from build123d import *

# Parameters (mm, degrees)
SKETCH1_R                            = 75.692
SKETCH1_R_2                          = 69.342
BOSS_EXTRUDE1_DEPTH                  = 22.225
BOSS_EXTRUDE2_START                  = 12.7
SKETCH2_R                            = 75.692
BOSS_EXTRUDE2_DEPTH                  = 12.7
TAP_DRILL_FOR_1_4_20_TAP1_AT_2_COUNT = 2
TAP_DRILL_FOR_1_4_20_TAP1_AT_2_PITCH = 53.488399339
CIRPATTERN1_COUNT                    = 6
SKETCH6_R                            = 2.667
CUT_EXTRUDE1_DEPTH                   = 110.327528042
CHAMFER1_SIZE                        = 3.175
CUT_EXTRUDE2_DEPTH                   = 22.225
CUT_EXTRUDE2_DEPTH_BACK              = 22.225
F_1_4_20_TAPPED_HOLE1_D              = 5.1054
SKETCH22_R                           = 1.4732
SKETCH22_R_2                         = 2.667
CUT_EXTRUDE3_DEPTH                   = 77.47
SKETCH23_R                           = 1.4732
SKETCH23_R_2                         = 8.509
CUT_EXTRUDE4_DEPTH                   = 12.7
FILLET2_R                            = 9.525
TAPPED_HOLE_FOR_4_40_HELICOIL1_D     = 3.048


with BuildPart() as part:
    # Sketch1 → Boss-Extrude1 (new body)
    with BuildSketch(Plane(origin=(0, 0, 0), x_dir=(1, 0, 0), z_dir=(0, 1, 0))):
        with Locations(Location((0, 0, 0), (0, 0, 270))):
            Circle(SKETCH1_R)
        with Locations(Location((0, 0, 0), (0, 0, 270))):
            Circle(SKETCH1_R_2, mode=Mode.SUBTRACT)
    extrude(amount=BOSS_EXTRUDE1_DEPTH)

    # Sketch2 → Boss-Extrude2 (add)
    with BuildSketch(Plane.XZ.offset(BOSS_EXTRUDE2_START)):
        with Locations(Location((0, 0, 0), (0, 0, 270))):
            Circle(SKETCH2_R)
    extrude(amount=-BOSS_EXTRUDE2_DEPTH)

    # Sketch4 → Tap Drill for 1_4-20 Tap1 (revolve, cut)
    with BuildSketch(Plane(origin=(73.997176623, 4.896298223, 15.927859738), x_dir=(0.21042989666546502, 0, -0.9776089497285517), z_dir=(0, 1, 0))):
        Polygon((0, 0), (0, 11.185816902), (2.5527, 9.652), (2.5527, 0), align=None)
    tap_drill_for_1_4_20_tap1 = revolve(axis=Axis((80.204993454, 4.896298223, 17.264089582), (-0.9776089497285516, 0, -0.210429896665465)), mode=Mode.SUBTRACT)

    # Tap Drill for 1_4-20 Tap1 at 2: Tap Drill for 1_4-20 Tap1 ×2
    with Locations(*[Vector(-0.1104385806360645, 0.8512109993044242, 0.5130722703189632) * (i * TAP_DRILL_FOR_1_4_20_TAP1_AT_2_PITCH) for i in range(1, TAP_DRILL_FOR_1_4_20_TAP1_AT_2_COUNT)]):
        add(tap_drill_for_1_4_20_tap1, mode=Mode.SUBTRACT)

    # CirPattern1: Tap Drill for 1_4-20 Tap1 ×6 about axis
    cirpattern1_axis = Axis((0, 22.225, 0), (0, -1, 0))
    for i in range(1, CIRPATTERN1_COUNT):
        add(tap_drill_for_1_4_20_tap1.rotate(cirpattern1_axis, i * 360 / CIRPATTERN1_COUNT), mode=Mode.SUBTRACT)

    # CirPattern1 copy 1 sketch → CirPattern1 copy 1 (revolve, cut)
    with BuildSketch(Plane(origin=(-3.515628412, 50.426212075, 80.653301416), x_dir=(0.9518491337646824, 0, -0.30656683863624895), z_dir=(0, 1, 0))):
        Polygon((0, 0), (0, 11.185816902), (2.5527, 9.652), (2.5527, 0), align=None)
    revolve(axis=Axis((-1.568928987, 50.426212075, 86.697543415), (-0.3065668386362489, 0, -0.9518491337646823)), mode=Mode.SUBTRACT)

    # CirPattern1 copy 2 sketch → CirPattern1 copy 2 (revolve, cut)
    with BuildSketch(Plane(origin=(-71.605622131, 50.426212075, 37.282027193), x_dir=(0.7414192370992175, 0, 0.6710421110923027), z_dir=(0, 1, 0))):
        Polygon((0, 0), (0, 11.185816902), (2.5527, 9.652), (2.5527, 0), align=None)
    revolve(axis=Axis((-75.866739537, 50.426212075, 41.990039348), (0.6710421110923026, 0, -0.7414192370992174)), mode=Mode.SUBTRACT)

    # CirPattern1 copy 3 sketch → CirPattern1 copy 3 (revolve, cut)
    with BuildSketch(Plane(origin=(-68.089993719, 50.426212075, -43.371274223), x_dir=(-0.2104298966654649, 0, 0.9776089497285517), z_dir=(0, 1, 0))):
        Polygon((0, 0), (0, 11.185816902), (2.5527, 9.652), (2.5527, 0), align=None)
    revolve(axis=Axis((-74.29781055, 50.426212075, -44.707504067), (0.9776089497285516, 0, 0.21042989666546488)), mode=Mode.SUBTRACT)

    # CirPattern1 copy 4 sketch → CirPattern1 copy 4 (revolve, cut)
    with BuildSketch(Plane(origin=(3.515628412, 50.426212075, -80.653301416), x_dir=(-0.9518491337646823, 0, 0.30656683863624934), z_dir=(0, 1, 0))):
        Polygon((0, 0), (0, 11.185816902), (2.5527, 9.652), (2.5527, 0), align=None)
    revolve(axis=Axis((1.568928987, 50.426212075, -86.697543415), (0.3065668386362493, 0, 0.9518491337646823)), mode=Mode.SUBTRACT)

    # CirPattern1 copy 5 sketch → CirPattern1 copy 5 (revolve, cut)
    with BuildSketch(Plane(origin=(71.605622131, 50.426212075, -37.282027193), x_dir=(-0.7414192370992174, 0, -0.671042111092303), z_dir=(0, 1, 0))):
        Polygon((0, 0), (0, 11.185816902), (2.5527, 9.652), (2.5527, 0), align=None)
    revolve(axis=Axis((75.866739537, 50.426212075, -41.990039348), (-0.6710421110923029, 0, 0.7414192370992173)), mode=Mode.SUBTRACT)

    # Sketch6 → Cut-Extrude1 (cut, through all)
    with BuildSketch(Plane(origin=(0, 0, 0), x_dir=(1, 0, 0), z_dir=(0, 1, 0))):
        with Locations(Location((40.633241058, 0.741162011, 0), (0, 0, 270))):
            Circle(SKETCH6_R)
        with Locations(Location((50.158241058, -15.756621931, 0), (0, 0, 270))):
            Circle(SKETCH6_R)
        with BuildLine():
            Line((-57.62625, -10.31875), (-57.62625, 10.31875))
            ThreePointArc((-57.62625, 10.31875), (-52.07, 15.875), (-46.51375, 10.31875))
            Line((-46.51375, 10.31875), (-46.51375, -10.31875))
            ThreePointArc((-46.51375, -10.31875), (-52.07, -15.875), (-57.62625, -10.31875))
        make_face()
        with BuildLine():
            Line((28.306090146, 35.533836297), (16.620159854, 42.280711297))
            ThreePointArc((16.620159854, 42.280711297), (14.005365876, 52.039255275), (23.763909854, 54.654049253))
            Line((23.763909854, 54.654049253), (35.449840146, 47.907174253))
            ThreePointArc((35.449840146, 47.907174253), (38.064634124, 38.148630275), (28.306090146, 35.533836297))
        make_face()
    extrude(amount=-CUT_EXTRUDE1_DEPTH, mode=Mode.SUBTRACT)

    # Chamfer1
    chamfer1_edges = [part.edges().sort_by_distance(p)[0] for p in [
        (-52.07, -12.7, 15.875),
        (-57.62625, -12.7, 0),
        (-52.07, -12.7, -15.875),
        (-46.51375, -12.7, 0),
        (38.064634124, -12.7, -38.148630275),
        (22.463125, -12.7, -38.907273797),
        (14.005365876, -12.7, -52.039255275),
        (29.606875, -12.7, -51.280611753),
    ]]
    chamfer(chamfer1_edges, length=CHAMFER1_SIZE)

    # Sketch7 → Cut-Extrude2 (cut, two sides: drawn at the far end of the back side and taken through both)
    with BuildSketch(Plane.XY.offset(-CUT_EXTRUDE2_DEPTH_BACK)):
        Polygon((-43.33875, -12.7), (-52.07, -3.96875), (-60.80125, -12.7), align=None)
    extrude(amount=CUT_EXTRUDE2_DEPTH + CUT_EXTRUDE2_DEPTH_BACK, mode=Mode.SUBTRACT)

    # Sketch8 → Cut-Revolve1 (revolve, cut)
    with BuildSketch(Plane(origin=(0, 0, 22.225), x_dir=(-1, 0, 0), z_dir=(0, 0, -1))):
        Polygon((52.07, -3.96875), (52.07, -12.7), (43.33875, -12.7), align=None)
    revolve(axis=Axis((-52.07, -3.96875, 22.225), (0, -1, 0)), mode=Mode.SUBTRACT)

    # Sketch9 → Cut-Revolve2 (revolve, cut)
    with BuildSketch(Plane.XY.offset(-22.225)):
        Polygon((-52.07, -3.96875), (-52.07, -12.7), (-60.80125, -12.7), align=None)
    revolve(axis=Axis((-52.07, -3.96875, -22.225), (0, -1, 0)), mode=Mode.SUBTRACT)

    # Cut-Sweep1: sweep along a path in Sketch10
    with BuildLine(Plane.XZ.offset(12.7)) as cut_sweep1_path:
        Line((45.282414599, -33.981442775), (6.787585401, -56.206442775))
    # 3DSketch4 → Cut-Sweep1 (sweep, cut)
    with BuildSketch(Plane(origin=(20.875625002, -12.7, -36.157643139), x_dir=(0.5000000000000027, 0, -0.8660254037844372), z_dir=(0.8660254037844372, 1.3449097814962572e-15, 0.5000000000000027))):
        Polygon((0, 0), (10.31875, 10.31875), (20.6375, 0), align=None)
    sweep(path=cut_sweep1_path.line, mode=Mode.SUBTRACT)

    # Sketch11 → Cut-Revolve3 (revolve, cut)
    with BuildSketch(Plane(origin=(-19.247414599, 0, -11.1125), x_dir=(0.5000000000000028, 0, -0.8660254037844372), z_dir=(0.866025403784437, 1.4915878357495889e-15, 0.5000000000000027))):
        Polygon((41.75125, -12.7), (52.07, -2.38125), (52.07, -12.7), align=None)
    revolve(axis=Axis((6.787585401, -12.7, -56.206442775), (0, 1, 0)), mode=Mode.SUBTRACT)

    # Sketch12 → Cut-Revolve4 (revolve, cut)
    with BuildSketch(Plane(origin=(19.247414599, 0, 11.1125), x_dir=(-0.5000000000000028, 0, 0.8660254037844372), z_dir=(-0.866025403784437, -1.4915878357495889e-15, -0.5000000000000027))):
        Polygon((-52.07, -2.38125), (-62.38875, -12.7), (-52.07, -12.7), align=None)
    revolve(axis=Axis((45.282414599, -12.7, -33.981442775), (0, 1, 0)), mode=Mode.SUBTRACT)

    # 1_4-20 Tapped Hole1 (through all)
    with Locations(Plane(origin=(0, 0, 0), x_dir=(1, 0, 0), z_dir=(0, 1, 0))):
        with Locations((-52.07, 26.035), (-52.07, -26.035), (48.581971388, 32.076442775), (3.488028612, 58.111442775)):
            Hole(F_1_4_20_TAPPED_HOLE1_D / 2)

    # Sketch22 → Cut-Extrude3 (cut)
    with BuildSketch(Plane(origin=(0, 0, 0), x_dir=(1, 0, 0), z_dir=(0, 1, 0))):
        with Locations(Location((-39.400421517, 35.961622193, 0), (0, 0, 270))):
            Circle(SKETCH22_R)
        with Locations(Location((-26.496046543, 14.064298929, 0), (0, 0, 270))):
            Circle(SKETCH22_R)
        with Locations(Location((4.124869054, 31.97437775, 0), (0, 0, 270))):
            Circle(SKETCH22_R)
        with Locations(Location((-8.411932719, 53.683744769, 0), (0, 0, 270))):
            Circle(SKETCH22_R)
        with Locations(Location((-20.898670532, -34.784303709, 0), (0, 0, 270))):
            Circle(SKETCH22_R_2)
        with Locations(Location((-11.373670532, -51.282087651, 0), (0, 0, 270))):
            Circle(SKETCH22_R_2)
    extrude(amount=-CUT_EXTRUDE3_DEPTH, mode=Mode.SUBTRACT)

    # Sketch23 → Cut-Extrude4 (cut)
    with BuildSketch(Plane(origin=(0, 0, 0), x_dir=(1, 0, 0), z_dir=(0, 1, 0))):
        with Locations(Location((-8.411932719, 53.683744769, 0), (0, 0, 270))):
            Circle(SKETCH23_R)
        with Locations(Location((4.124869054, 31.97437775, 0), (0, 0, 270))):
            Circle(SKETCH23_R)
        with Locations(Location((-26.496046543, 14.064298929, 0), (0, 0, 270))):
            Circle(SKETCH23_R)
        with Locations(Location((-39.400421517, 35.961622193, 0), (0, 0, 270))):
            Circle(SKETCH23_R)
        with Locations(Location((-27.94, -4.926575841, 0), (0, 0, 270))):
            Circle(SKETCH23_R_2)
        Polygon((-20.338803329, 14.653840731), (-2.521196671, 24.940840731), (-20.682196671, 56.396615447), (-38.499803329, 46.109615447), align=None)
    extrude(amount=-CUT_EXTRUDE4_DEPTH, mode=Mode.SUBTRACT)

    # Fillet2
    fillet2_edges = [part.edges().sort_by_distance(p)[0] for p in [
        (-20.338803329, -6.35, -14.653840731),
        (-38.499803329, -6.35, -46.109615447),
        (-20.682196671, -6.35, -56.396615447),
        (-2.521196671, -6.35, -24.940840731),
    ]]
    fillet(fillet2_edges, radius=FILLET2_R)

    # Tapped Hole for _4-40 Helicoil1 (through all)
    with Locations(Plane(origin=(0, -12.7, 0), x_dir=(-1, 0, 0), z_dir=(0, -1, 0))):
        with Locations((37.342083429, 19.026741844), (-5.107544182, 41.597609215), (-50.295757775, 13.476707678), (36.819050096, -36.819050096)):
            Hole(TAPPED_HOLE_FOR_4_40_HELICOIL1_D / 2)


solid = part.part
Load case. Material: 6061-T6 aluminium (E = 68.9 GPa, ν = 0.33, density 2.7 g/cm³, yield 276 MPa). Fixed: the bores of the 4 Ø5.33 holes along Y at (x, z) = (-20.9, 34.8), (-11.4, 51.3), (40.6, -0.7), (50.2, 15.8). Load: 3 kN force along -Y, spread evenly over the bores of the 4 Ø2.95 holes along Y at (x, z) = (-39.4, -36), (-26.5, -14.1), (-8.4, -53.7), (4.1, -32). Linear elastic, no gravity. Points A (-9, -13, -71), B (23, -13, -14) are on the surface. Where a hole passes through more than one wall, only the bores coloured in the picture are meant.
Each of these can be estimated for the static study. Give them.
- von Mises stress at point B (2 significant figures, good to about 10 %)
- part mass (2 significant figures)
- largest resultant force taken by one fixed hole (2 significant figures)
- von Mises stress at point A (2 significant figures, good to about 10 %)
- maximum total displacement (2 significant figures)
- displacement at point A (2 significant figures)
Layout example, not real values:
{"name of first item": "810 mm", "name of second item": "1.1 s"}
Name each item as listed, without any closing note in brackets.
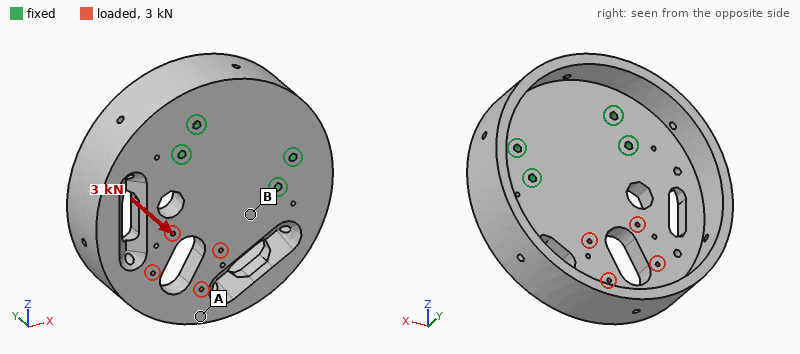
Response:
{"von Mises stress at point B": "21 MPa", "part mass": "710 g", "largest resultant force taken by one fixed hole": "3.7 kN", "von Mises stress at point A": "9.6 MPa", "maximum total displacement": "0.24 mm", "displacement at point A": "0.19 mm"}
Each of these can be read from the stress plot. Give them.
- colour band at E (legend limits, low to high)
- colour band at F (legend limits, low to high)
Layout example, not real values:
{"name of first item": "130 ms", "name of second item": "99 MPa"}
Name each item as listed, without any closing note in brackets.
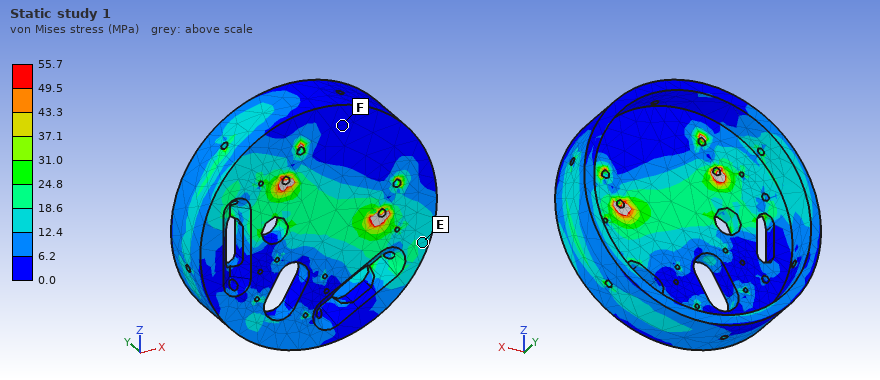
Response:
{"colour band at E": "12.4 to 18.6 MPa", "colour band at F": "0.0 to 6.2 MPa"}
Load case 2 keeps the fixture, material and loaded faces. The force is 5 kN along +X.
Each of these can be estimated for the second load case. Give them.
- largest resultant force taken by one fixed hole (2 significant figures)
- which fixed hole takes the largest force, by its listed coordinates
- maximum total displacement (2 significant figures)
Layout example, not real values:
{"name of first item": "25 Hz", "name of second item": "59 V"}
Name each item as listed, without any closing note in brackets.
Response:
{"largest resultant force taken by one fixed hole": "4.0 kN", "which fixed hole takes the largest force, by its listed coordinates": "(40.6, -0.7)", "maximum total displacement": "20 µm"}
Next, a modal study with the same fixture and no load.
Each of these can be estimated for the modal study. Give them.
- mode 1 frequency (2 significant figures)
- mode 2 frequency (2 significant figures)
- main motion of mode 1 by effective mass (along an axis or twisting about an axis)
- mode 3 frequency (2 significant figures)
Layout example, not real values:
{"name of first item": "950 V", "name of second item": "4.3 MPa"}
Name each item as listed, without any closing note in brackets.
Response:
{"mode 1 frequency": "1300 Hz", "mode 2 frequency": "2300 Hz", "main motion of mode 1 by effective mass": "along Y", "mode 3 frequency": "3500 Hz"}
